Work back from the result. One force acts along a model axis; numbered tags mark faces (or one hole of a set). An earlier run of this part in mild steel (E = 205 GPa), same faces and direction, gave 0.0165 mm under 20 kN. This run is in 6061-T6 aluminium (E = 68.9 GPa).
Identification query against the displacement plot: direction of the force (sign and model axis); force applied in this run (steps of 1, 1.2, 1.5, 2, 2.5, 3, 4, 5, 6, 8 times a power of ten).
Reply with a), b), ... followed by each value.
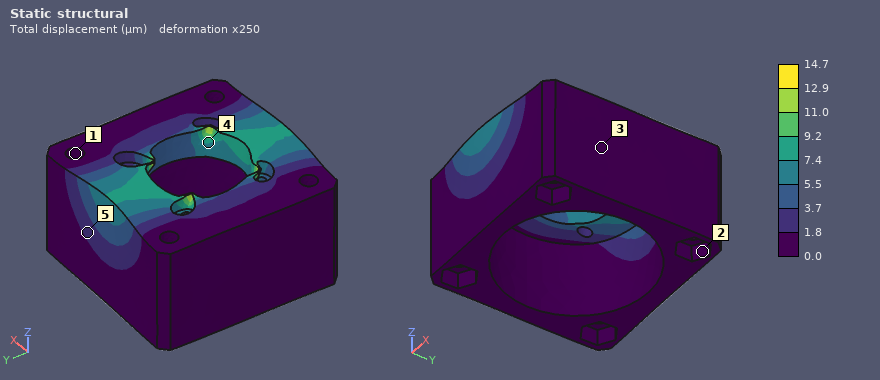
a) -Y
b) 6 kN
